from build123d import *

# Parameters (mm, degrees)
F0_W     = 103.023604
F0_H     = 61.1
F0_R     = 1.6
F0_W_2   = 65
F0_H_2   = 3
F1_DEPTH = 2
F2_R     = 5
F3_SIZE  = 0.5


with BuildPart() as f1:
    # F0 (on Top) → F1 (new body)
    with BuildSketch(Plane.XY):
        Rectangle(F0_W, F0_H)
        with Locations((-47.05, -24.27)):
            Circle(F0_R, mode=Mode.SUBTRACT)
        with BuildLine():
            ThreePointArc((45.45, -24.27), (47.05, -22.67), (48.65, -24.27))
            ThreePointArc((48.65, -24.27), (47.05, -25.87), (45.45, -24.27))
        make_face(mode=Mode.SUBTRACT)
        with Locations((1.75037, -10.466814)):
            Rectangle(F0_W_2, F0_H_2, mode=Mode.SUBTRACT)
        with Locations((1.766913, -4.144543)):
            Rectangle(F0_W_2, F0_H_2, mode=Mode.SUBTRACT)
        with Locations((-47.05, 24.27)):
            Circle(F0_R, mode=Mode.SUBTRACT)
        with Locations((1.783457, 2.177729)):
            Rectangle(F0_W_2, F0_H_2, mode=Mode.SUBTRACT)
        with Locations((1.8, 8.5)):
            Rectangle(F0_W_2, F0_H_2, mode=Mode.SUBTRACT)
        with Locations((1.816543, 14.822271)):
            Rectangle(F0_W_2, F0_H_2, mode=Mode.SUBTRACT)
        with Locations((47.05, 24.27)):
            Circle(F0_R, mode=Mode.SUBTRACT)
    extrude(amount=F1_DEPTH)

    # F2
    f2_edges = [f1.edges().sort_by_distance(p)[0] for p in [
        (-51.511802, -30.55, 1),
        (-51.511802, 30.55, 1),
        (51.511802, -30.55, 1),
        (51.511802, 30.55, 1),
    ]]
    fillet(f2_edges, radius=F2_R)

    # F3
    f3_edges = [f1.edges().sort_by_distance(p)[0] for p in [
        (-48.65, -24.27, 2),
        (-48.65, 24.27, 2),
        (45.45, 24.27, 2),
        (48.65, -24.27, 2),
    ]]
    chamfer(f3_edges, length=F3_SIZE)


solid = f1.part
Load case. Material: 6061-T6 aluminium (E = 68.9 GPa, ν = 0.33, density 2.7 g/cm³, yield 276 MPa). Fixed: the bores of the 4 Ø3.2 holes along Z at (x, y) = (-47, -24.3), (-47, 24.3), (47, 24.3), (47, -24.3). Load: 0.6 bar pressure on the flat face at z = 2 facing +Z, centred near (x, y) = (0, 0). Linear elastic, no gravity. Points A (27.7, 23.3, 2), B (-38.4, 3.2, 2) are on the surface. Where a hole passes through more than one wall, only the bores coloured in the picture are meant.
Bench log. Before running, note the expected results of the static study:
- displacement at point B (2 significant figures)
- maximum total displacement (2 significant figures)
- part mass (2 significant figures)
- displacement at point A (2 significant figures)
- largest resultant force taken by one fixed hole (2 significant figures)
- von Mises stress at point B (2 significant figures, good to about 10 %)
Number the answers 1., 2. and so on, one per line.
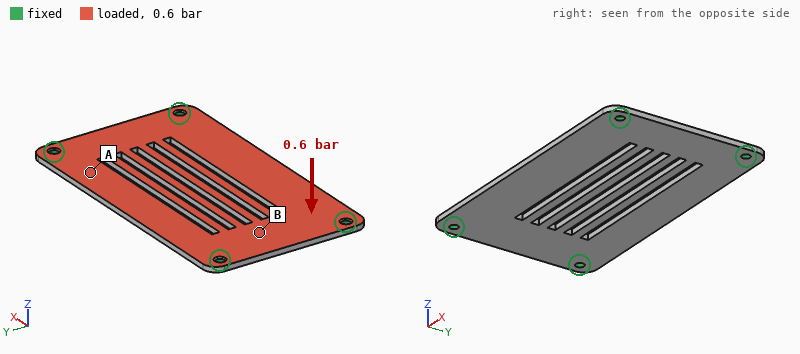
1. 0.099 mm
2. 0.39 mm
3. 28 g
4. 0.14 mm
5. 84 N
6. 22 MPa
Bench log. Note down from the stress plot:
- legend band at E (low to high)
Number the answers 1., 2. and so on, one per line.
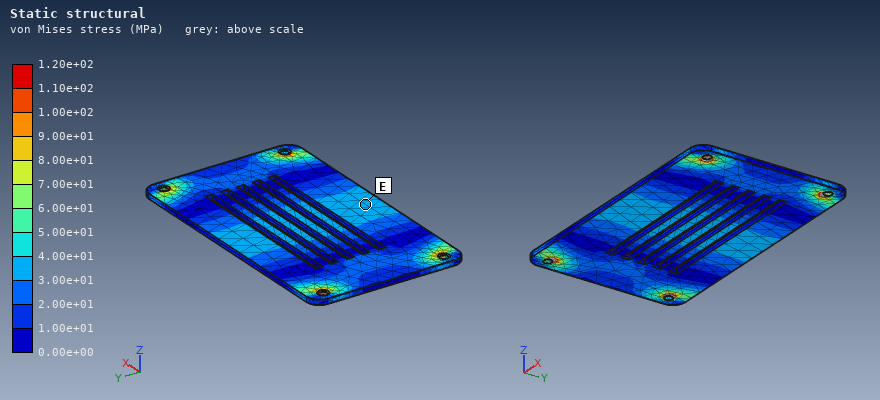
1. 3.00e+01 to 4.00e+01 MPa
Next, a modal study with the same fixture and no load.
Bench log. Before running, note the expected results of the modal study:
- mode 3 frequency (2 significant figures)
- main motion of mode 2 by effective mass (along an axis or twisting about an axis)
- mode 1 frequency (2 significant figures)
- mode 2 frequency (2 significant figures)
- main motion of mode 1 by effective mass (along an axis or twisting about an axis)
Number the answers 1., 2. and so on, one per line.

1. 1600 Hz
2. twisting about X
3. 1100 Hz
4. 1300 Hz
5. along Z
